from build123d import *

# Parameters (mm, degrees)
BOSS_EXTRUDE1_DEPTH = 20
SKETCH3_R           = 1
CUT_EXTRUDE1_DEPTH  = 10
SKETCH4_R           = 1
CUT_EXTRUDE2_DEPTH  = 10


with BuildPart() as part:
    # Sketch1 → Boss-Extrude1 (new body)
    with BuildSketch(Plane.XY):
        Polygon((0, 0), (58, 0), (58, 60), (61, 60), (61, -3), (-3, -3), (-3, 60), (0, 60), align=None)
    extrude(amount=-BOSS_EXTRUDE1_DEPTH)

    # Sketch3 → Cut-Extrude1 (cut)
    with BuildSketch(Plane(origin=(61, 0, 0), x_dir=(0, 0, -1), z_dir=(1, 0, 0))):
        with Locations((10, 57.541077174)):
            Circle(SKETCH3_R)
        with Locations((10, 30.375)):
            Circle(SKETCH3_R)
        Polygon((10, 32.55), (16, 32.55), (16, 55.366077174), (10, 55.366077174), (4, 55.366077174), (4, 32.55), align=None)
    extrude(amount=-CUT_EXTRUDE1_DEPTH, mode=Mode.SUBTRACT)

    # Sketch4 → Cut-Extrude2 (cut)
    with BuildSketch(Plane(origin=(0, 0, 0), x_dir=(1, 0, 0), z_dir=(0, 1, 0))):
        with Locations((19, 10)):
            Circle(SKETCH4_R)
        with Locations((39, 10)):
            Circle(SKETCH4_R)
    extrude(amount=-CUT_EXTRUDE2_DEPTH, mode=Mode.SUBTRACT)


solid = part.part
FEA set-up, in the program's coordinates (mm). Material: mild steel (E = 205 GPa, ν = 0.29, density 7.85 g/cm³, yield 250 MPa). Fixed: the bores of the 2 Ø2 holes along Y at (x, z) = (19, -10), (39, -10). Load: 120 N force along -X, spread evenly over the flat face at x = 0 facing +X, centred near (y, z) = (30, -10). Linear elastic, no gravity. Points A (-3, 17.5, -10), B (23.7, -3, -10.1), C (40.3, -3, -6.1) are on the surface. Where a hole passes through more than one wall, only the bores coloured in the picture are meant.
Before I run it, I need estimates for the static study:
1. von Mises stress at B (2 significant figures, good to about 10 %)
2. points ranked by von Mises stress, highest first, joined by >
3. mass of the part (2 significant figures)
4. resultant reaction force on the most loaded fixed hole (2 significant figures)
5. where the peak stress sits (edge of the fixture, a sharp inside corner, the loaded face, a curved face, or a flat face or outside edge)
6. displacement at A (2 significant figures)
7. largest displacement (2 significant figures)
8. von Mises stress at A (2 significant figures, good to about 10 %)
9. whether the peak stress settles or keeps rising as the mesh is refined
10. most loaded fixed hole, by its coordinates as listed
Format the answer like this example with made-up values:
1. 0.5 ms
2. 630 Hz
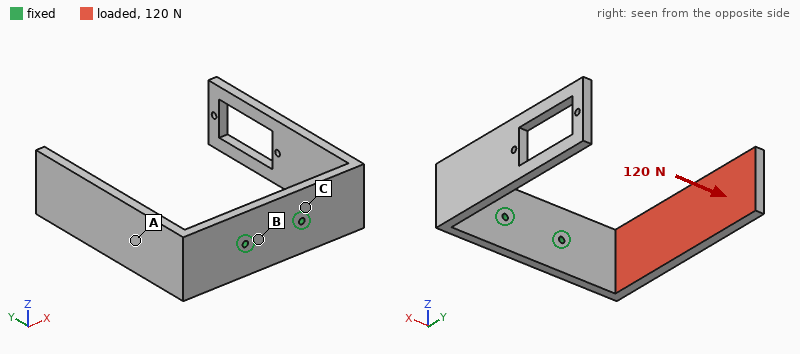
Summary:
1. 30 MPa
2. A > B > C
3. 80 g
4. 120 N
5. edge of the fixture
6. 0.24 mm
7. 0.89 mm
8. 58 MPa
9. keeps rising
10. (19, -10)
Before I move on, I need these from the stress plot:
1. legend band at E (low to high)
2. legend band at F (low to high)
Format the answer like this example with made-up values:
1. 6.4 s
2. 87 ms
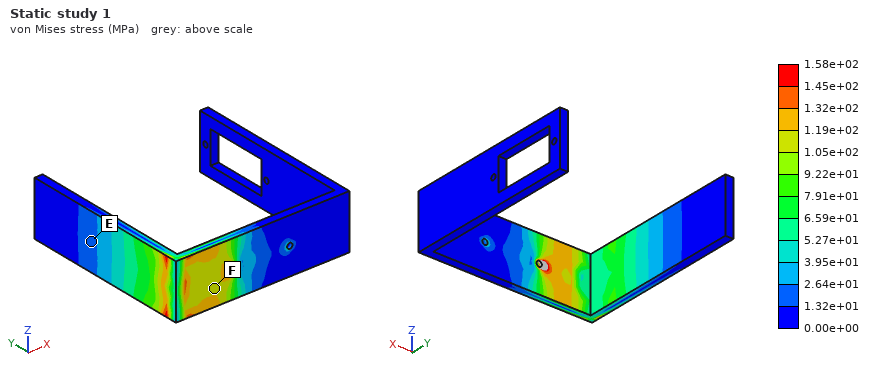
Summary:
1. 1.32e+01 to 2.64e+01 MPa
2. 1.05e+02 to 1.19e+02 MPa
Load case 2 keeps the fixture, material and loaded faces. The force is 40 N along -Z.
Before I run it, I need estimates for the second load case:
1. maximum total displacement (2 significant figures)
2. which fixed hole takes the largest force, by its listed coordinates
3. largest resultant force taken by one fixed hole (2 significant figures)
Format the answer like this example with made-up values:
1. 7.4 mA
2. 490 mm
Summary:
1. 0.12 mm
2. (19, -10)
3. 74 N
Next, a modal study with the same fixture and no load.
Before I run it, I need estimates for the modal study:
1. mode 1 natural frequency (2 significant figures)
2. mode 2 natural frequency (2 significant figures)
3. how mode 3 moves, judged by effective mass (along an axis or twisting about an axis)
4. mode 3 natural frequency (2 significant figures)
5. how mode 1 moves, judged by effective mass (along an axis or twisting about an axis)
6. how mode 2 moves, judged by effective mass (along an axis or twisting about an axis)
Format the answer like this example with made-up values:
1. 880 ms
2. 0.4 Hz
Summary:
1. 420 Hz
2. 540 Hz
3. along Z
4. 660 Hz
5. along X
6. along X
